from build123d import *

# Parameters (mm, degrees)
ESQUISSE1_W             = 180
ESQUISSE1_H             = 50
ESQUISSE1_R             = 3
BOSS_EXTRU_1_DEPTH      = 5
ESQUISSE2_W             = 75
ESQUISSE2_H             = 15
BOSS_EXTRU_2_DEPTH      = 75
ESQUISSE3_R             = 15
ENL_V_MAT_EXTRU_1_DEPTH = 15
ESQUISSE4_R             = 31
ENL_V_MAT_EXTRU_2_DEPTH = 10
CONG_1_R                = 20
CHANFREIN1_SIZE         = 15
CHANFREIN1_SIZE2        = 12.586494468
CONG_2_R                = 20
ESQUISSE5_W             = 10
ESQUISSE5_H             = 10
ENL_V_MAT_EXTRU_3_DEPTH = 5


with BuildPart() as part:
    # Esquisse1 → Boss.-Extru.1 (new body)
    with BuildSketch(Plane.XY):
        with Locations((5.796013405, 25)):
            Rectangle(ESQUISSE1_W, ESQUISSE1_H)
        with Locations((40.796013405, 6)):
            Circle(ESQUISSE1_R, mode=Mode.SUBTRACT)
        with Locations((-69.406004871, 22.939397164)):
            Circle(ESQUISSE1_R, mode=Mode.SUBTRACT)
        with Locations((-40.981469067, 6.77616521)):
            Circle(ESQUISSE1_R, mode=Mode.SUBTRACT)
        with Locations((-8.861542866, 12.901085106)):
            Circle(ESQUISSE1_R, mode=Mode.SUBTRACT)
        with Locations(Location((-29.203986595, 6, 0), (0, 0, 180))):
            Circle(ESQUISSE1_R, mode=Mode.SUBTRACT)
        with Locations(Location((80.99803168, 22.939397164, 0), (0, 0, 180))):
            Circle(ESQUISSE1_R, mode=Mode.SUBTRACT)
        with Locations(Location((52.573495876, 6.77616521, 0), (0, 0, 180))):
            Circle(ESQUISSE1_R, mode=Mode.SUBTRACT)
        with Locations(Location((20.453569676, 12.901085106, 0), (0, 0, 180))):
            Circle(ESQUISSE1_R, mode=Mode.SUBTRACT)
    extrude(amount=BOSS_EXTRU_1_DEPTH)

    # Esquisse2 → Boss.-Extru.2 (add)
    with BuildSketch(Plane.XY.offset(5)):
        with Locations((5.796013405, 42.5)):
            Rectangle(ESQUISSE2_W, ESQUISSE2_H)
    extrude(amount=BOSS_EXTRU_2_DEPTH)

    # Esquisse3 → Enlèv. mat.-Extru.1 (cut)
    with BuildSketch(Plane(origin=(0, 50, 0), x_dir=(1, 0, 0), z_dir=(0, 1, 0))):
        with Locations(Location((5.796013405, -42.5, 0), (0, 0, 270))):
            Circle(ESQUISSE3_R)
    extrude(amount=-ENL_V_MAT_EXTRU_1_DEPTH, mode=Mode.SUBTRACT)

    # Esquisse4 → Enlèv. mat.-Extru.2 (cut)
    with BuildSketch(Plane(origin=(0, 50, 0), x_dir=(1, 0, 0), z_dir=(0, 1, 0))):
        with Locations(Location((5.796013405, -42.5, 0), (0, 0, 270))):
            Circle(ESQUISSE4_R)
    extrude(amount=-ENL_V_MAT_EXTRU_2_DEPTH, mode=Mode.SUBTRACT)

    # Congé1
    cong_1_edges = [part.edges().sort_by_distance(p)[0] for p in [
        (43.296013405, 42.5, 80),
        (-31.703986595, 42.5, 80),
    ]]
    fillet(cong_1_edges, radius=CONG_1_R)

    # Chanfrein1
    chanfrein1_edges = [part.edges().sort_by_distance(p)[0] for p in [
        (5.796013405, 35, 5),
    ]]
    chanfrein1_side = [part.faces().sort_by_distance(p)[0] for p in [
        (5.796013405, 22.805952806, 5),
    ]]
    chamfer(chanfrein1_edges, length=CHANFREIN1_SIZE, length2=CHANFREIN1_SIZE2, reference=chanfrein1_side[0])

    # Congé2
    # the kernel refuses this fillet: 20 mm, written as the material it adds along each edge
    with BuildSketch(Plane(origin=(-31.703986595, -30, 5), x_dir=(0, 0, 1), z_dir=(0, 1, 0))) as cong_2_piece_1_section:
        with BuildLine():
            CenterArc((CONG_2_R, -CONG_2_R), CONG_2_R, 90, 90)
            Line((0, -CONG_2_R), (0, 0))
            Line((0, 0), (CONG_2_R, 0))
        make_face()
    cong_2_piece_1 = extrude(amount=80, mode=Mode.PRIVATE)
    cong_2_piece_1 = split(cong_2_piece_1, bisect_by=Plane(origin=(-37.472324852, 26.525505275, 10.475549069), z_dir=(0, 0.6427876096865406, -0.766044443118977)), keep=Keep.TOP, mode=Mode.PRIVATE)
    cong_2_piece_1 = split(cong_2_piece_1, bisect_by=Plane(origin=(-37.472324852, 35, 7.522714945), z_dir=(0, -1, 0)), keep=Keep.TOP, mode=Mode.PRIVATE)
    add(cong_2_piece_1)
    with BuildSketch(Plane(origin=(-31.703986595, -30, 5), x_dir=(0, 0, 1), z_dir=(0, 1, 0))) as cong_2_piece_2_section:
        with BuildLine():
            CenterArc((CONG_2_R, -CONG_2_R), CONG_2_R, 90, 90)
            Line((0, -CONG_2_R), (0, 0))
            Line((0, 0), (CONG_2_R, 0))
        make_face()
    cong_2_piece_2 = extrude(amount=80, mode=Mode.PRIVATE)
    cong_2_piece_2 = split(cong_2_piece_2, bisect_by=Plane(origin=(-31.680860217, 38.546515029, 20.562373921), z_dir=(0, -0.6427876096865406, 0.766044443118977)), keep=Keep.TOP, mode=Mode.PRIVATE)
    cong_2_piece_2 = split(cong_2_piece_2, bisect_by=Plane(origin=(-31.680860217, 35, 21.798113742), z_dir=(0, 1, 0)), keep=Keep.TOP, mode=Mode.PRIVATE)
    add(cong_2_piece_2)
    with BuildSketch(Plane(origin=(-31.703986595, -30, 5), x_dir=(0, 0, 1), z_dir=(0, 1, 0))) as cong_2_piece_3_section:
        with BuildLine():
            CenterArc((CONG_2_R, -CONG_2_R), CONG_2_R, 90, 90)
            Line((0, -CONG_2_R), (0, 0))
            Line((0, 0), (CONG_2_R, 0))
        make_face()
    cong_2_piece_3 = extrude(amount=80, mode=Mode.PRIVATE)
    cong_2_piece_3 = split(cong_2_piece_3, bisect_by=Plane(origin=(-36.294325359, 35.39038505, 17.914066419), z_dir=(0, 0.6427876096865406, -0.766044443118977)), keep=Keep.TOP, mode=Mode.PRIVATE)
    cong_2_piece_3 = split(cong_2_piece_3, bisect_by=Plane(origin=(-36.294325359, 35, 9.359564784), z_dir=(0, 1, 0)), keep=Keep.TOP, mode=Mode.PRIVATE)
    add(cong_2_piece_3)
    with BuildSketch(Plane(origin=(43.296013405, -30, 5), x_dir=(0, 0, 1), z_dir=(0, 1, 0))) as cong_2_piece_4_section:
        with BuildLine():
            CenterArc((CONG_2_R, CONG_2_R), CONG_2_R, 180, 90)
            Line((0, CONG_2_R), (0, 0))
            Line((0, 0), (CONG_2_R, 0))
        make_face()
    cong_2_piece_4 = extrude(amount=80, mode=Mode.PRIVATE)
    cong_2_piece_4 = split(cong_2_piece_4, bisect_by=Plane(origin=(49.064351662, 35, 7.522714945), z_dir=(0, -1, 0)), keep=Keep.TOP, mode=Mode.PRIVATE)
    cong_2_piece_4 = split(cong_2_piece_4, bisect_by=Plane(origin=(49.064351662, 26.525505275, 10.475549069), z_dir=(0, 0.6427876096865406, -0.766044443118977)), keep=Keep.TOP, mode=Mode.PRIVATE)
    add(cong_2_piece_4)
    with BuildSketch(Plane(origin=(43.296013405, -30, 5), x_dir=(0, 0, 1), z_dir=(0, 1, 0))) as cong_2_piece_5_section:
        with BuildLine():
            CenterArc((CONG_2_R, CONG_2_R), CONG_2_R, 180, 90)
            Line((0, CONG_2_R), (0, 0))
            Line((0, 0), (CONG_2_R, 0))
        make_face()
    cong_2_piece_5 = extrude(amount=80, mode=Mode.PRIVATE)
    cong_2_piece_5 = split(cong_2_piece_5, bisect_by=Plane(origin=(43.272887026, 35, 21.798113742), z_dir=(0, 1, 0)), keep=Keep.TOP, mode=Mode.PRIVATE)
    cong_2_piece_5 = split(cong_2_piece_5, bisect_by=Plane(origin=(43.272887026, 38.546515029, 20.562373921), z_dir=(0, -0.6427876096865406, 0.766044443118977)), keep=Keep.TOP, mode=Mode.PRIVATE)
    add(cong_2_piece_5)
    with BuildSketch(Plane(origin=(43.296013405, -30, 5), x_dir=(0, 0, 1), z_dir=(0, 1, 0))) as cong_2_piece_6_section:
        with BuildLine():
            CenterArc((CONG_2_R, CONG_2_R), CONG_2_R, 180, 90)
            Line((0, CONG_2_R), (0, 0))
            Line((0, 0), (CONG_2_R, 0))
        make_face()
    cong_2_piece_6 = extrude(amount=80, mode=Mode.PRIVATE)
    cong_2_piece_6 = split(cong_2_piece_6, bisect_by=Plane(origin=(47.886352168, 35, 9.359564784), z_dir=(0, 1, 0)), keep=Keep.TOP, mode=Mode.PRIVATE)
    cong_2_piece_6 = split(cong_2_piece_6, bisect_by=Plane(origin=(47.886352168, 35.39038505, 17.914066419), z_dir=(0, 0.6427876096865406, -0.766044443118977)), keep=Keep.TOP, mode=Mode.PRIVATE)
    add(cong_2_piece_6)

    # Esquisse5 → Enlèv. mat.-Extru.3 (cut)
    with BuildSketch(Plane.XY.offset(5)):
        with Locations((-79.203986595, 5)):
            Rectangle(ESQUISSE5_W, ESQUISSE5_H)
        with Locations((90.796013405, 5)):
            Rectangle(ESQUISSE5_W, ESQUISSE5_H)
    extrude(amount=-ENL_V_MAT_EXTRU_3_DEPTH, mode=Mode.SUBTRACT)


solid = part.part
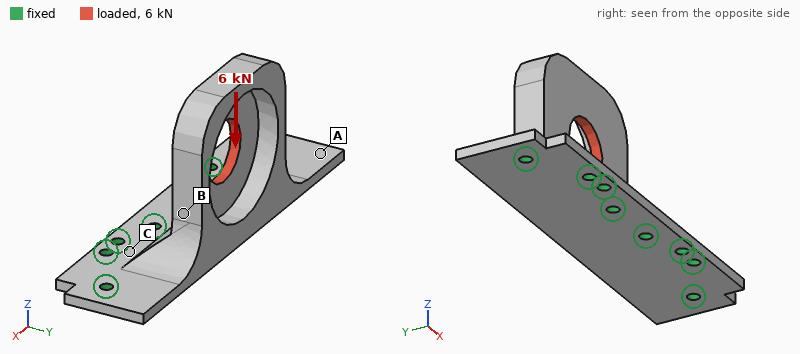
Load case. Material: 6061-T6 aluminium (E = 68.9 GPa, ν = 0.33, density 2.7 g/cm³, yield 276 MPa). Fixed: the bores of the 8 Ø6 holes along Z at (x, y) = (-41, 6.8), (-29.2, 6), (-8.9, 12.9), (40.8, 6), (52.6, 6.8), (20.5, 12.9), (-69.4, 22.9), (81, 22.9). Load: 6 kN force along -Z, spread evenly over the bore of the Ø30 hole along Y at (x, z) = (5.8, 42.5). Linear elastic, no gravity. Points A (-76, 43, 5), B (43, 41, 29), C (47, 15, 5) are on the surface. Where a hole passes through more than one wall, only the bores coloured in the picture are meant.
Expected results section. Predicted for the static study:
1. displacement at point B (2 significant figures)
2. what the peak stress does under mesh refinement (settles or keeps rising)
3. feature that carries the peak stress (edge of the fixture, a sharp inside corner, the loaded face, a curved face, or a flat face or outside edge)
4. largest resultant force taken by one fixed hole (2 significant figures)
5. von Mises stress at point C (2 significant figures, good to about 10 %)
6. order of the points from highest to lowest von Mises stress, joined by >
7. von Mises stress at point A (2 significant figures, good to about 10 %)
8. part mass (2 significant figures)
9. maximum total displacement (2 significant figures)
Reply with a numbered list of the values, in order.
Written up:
1. 0.36 mm
2. keeps rising
3. edge of the fixture
4. 2.1 kN
5. 110 MPa
6. C > A > B
7. 44 MPa
8. 280 g
9. 0.82 mm
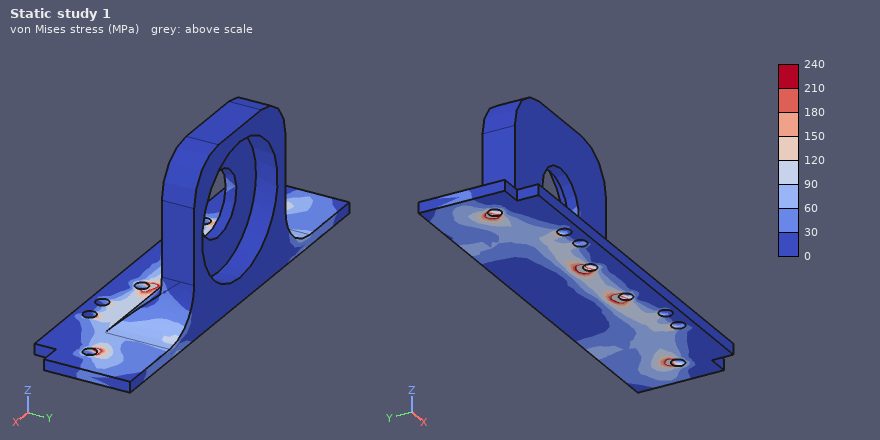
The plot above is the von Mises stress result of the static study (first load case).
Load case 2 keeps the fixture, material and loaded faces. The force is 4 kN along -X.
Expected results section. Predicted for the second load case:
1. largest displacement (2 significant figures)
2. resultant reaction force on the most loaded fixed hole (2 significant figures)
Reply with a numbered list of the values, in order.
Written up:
1. 0.14 mm
2. 1.1 kN
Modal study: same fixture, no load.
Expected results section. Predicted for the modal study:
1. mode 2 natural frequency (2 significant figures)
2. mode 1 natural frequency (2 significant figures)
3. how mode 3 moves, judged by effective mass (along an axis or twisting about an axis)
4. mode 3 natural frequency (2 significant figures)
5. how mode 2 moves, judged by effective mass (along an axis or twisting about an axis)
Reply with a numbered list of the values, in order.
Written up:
1. 2400 Hz
2. 820 Hz
3. along Z
4. 3300 Hz
5. along X
